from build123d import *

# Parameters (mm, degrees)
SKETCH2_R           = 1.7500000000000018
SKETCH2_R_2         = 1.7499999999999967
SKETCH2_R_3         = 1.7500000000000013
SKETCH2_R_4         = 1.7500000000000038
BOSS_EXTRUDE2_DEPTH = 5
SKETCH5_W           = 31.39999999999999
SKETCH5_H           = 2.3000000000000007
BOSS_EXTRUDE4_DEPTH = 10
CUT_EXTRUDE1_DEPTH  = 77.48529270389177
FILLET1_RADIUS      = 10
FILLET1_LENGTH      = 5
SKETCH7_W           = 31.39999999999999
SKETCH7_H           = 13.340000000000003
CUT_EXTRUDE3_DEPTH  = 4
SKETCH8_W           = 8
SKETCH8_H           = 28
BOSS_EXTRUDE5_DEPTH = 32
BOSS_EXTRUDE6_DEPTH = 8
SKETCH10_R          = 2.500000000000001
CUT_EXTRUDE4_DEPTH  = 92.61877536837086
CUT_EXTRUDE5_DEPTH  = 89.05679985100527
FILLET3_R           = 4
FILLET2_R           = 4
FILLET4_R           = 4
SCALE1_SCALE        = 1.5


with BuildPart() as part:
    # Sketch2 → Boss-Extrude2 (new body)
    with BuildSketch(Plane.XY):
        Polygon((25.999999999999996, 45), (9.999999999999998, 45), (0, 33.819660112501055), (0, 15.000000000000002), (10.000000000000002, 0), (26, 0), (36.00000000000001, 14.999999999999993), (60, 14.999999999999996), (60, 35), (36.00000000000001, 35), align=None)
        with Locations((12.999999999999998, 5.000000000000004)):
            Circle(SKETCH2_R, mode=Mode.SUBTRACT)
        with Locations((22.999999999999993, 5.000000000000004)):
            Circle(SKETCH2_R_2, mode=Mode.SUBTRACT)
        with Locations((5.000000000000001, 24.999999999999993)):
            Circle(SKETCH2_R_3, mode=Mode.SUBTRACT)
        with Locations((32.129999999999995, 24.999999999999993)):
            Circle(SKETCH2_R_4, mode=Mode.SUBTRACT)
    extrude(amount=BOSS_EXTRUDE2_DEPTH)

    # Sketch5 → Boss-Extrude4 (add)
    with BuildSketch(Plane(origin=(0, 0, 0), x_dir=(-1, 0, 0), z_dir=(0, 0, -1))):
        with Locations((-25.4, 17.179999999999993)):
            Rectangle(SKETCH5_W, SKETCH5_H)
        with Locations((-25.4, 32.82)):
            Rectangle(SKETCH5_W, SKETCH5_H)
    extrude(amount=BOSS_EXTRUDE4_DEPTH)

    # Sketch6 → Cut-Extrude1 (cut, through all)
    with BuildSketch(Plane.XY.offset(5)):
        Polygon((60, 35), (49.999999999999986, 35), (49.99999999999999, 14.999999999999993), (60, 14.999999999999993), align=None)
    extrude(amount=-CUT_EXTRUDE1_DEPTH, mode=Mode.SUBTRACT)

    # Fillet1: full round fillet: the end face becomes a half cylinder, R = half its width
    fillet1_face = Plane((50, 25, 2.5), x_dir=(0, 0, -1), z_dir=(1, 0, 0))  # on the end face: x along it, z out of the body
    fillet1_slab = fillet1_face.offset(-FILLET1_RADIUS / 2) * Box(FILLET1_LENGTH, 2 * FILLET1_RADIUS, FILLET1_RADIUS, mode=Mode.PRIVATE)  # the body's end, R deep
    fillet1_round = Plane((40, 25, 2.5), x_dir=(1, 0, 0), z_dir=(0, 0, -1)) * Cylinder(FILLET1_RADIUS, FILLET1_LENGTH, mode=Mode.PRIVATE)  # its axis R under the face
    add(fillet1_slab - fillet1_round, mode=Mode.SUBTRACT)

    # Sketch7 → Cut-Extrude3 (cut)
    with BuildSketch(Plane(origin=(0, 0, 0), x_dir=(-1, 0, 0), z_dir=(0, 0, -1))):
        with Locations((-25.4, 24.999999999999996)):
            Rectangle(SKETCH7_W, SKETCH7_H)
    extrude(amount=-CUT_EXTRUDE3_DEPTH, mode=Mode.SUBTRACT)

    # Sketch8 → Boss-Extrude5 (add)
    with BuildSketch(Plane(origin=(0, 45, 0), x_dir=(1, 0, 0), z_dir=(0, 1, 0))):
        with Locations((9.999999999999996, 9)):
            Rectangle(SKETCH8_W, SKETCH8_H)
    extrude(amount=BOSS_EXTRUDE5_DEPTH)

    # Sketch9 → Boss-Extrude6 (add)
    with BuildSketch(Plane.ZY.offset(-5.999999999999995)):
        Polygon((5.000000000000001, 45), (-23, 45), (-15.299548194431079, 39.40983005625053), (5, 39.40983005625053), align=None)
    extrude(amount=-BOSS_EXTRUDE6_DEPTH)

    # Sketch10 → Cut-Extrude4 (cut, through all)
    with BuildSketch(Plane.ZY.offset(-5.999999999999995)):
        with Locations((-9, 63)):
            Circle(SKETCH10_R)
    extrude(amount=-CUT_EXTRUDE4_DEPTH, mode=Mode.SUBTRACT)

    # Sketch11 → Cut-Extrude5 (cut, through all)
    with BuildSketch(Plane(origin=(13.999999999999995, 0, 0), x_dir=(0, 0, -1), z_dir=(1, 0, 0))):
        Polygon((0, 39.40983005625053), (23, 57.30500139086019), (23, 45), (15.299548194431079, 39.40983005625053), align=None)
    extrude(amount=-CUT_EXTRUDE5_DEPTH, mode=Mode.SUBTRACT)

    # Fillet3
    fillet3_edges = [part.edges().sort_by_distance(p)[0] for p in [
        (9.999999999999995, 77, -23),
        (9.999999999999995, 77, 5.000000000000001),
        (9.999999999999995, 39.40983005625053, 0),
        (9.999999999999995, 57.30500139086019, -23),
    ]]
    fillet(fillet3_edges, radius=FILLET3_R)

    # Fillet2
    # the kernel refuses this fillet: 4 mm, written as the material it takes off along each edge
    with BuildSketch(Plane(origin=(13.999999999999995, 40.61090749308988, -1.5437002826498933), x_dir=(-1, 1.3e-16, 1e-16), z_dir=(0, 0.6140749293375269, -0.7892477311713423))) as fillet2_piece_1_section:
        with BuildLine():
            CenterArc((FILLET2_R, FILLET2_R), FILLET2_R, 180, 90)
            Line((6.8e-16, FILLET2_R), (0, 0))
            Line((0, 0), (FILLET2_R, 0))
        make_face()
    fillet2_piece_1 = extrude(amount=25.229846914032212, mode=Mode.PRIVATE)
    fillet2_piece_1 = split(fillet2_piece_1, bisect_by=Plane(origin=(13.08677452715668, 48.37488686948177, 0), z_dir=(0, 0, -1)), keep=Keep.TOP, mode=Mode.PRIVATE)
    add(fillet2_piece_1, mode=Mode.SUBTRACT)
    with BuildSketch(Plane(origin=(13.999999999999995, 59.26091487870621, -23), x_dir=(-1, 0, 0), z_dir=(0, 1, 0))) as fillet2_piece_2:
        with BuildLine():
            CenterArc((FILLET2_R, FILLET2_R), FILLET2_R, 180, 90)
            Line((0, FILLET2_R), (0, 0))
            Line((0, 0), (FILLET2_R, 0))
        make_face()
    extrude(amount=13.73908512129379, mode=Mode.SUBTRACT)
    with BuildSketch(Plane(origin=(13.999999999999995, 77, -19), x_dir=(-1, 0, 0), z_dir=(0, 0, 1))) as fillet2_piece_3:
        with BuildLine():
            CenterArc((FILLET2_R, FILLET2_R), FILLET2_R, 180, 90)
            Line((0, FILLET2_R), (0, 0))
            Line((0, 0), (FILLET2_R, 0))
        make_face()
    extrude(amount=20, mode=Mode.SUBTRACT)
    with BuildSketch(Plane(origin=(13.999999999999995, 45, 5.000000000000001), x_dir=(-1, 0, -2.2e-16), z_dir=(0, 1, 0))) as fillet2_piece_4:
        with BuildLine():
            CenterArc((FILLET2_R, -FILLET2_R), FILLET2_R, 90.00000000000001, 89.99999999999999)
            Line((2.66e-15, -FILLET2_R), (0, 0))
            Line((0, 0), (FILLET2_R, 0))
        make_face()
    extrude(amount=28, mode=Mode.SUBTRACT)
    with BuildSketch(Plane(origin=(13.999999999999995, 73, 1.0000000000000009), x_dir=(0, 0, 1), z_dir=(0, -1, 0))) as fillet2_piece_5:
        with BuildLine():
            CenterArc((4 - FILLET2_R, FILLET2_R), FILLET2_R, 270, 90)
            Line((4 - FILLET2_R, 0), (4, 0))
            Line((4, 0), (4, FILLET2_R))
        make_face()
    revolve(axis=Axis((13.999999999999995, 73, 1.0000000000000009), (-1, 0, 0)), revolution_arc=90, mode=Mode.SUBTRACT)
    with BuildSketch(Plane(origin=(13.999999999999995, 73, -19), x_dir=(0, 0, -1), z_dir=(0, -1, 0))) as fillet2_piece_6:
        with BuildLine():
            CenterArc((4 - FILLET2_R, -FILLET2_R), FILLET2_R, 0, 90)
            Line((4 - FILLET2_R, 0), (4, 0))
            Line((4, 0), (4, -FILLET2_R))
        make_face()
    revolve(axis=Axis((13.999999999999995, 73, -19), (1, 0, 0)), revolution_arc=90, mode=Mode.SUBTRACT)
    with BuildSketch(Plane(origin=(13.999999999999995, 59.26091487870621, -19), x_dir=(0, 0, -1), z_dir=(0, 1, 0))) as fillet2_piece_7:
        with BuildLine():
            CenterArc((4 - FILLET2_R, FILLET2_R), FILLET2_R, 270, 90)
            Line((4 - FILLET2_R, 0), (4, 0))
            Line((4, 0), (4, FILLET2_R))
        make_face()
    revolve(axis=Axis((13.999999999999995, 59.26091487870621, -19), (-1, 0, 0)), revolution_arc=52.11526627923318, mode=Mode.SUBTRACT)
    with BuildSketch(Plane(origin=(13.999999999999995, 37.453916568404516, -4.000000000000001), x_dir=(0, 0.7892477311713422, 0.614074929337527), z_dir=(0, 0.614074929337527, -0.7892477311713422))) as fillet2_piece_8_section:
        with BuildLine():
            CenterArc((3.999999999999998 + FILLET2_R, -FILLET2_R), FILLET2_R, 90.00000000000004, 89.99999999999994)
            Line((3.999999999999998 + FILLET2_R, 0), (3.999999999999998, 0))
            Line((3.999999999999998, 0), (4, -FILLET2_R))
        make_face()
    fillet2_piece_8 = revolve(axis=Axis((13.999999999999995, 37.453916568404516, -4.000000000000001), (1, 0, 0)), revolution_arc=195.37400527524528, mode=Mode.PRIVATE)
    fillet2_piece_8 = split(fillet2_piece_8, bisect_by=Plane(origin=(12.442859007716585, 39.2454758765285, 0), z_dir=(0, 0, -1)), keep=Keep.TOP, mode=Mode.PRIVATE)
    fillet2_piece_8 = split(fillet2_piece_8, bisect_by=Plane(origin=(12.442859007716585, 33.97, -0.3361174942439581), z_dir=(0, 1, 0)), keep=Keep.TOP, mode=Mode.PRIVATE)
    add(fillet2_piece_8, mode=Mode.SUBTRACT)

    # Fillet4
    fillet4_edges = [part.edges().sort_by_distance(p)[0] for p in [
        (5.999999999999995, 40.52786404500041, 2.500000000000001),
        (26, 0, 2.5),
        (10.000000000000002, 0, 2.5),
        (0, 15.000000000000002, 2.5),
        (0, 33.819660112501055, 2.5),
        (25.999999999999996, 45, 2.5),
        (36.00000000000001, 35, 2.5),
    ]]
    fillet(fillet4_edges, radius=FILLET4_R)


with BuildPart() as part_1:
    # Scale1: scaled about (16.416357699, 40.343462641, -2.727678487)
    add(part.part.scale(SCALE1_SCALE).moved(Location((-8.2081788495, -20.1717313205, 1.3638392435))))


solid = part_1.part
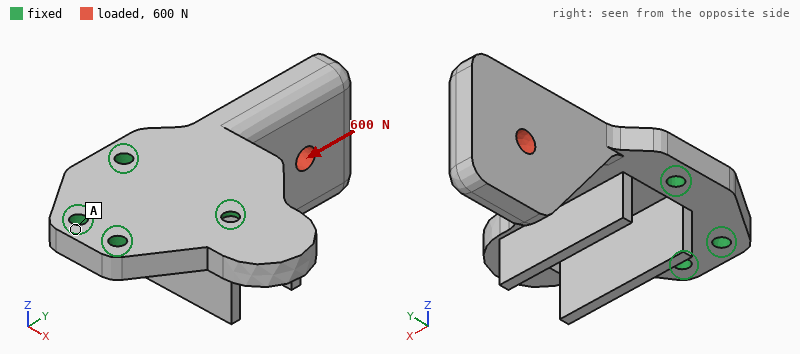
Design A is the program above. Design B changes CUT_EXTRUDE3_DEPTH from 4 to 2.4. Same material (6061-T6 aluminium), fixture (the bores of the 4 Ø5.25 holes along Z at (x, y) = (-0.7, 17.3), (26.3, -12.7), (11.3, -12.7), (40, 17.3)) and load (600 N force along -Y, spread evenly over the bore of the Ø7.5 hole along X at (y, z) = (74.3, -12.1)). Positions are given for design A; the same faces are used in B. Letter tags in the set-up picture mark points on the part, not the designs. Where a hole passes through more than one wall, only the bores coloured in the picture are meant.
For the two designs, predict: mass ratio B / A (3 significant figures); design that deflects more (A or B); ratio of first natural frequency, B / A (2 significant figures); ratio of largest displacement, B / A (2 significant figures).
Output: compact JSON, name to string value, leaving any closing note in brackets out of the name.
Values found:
{"mass ratio B / A": "1.05", "design that deflects more": "A", "ratio of first natural frequency, B / A": "1.1", "ratio of largest displacement, B / A": "0.84"}
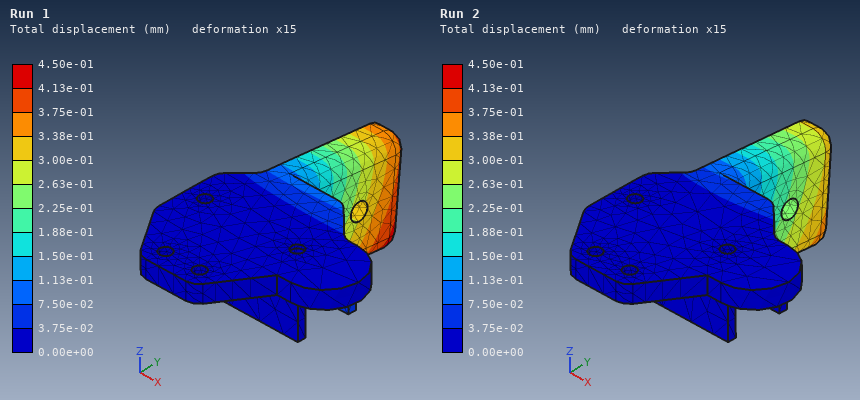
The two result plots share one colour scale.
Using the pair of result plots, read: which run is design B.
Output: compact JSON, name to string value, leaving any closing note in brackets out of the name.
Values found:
{"which run is design B": "Run 2"}
